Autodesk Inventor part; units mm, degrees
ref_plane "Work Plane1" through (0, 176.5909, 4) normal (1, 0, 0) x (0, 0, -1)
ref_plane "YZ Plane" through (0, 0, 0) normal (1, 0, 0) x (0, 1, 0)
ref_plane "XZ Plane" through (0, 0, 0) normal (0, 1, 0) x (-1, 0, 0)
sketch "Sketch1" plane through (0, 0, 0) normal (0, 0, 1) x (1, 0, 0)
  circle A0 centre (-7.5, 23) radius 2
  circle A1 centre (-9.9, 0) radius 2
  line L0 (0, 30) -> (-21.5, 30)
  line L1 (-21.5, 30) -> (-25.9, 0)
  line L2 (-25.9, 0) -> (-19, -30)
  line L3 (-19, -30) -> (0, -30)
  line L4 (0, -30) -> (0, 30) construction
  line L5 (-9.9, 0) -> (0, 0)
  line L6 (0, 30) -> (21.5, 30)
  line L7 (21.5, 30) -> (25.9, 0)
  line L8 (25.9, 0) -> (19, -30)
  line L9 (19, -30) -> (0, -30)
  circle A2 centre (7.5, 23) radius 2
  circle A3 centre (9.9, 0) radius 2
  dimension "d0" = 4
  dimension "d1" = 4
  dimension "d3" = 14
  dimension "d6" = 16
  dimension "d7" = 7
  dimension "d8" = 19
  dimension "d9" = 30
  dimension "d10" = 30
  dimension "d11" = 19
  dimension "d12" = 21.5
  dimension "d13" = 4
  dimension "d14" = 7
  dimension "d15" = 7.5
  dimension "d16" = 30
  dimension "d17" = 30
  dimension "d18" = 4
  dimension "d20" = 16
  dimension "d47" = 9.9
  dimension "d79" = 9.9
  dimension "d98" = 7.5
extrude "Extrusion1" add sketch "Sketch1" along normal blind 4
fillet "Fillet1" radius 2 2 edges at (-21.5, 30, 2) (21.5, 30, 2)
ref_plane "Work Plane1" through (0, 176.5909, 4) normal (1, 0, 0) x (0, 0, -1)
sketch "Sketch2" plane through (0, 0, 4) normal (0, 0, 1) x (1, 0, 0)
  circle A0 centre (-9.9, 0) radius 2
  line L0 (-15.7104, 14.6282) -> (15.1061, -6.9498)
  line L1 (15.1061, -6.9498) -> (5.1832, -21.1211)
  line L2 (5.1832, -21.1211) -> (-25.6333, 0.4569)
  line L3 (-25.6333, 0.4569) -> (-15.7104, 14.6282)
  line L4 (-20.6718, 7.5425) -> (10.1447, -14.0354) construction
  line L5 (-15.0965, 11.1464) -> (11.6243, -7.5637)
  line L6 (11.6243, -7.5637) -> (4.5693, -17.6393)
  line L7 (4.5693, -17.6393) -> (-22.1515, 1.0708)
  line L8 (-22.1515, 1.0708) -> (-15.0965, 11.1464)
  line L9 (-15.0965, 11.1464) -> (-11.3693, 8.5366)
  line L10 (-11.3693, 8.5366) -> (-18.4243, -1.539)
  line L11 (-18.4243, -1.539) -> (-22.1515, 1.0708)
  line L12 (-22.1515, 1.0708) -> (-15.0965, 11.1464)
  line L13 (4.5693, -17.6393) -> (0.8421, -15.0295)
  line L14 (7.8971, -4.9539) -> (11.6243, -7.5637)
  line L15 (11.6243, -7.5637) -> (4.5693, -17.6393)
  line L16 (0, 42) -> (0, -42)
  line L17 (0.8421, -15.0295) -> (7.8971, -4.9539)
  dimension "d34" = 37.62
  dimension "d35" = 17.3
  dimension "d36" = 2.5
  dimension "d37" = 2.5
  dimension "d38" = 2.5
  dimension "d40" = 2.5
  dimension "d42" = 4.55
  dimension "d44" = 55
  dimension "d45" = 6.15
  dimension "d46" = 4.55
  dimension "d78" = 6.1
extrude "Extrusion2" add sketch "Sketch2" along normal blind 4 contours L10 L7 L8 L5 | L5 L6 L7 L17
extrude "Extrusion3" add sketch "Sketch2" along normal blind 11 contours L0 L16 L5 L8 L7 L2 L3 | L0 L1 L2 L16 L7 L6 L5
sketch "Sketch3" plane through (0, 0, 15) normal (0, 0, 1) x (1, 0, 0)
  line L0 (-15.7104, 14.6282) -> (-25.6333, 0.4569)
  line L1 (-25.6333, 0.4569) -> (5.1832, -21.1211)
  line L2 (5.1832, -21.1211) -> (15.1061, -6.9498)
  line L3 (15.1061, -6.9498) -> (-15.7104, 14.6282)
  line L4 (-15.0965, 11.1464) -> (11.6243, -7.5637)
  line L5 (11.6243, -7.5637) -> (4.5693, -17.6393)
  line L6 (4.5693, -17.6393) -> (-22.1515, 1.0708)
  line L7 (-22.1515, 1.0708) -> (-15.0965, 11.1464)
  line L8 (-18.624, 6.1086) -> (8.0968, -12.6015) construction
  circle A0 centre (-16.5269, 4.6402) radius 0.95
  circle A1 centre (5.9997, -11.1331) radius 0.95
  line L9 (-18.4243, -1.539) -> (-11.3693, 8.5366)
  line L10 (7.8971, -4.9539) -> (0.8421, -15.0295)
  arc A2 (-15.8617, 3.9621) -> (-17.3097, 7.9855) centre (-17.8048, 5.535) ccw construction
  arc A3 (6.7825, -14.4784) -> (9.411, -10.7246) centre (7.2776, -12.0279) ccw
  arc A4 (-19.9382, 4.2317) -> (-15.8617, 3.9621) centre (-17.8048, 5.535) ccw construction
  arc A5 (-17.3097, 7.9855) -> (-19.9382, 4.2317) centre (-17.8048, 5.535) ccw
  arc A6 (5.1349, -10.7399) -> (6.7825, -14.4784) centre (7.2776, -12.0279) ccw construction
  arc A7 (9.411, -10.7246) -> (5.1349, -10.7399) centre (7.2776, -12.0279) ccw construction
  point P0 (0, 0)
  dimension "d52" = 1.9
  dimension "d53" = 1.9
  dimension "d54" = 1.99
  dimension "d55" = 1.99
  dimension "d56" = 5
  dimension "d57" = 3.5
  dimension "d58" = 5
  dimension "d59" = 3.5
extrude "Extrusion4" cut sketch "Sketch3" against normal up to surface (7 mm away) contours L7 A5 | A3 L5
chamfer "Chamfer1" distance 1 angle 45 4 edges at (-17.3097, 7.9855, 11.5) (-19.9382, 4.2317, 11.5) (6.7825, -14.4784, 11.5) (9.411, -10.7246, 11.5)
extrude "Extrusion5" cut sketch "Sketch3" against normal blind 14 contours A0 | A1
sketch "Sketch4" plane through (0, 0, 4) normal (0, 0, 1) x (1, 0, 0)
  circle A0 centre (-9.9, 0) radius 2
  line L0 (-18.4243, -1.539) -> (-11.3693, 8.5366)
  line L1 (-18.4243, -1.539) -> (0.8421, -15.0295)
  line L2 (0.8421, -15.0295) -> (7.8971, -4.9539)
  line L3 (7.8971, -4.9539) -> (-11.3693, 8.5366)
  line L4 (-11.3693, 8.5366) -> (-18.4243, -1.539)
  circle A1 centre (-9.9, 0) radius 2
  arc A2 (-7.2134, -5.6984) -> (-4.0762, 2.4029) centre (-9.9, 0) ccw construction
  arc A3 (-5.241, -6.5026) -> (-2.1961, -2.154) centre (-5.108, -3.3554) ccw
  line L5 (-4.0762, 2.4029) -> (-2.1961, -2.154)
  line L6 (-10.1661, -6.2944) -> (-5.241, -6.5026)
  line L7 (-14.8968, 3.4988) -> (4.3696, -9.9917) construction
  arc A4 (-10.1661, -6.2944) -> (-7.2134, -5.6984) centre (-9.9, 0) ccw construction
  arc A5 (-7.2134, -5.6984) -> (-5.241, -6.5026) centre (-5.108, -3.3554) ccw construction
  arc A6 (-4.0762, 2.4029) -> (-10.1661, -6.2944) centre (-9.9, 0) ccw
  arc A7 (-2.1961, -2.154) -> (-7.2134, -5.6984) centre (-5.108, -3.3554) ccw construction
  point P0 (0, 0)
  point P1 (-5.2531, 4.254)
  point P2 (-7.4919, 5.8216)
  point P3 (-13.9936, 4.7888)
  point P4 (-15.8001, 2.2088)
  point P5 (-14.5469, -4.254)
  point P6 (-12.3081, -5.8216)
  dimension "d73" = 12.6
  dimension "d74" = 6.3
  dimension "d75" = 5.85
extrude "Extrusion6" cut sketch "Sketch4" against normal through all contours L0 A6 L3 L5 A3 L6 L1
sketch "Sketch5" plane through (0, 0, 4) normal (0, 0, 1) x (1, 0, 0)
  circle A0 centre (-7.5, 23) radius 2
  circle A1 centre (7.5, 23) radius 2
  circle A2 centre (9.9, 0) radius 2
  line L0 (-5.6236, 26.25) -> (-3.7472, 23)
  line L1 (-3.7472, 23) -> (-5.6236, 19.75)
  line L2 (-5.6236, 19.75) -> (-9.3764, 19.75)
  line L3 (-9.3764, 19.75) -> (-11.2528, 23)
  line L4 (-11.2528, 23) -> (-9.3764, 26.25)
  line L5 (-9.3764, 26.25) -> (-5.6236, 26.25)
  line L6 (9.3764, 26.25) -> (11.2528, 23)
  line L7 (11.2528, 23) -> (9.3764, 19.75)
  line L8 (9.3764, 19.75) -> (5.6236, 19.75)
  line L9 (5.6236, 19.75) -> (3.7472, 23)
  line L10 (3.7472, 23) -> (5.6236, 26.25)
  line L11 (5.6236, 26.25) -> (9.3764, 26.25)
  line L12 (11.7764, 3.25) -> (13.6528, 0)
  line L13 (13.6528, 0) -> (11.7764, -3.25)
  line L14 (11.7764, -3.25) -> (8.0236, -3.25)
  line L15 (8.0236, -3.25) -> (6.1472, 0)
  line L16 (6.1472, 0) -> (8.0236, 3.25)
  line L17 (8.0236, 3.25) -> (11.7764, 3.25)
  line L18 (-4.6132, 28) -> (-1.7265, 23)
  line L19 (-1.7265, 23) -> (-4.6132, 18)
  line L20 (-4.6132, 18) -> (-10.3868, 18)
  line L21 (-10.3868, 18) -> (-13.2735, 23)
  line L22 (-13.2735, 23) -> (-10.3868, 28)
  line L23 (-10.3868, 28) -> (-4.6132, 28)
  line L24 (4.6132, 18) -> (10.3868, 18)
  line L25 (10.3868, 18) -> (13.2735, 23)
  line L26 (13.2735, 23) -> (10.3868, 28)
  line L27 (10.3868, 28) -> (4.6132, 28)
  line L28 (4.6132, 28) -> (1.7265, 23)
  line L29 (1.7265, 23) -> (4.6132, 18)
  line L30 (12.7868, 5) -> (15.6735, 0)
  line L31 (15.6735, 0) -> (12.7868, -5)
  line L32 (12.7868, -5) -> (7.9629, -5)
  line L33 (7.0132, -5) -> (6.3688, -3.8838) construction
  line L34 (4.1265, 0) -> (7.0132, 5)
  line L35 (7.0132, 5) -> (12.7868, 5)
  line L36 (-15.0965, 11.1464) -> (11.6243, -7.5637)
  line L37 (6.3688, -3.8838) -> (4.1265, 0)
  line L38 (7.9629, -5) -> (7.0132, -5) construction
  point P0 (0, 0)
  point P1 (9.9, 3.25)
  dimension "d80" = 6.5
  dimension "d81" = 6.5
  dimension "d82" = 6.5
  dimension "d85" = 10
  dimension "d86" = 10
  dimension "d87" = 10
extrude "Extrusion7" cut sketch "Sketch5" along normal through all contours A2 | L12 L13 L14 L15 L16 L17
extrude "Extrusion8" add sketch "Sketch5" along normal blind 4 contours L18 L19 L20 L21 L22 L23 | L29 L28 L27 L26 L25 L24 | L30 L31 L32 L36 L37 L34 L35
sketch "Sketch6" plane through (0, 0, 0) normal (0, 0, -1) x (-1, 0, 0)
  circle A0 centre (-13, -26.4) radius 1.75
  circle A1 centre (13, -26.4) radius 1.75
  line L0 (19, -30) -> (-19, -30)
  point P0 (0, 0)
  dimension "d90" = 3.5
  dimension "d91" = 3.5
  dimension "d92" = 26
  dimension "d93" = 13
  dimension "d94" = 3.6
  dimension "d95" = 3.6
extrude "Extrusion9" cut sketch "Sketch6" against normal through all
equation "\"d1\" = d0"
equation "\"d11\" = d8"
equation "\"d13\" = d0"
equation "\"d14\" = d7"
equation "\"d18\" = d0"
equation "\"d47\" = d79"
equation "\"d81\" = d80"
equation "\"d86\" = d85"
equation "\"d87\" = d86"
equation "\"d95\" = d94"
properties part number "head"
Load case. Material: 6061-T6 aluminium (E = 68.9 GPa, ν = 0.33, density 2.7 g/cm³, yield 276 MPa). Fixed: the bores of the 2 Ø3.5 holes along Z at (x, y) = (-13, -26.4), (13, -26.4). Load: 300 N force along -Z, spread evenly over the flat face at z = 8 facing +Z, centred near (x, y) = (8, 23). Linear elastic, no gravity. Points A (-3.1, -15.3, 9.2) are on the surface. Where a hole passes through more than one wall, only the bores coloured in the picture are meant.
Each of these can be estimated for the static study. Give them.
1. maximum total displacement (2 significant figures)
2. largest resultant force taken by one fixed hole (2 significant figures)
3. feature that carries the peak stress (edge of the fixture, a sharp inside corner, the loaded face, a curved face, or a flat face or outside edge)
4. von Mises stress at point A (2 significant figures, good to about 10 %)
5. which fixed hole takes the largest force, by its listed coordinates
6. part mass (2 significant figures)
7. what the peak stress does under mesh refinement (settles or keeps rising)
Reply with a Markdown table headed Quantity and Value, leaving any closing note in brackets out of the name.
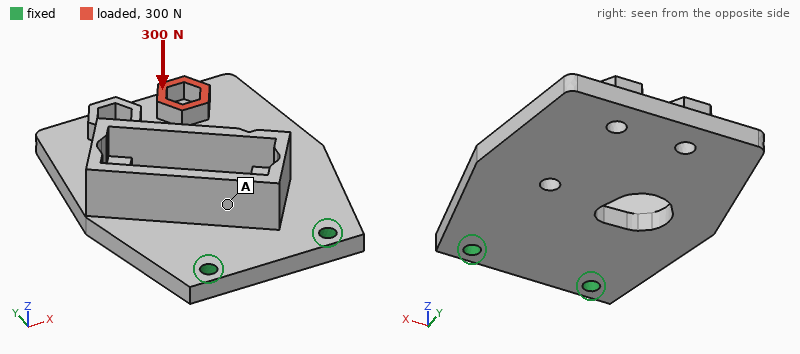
| Quantity | Value |
|---|---|
| maximum total displacement | 0.81 mm |
| largest resultant force taken by one fixed hole | 220 N |
| feature that carries the peak stress | edge of the fixture |
| von Mises stress at point A | 23 MPa |
| which fixed hole takes the largest force, by its listed coordinates | (13, -26.4) |
| part mass | 37 g |
| what the peak stress does under mesh refinement | keeps rising |
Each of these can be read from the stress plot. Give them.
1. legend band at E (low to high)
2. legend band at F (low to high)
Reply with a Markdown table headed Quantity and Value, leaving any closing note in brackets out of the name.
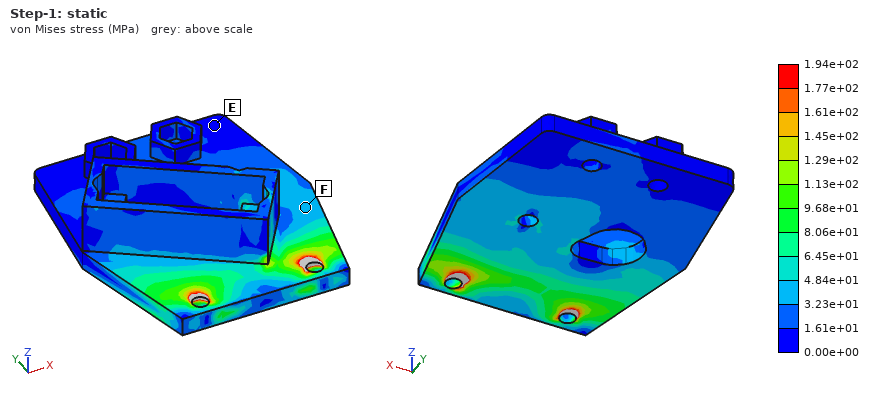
| Quantity | Value |
|---|---|
| legend band at E | 0.00e+00 to 1.61e+01 MPa |
| legend band at F | 3.23e+01 to 4.84e+01 MPa |
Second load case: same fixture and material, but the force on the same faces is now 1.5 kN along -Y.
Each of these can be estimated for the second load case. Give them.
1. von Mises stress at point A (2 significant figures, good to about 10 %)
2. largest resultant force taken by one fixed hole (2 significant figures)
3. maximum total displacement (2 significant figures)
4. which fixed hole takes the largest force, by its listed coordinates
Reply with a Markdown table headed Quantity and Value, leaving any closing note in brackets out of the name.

| Quantity | Value |
|---|---|
| von Mises stress at point A | 23 MPa |
| largest resultant force taken by one fixed hole | 1.2 kN |
| maximum total displacement | 0.72 mm |
| which fixed hole takes the largest force, by its listed coordinates | (13, -26.4) |
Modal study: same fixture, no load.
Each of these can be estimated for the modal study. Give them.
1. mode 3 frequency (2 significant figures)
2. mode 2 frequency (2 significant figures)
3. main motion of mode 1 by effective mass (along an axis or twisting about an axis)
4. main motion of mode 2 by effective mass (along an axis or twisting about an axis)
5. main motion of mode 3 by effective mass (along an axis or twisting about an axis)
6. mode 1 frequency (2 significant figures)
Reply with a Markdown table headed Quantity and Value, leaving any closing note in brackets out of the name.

| Quantity | Value |
|---|---|
| mode 3 frequency | 5700 Hz |
| mode 2 frequency | 3400 Hz |
| main motion of mode 1 by effective mass | along Z |
| main motion of mode 2 by effective mass | twisting about Y |
| main motion of mode 3 by effective mass | along X |
| mode 1 frequency | 970 Hz |
